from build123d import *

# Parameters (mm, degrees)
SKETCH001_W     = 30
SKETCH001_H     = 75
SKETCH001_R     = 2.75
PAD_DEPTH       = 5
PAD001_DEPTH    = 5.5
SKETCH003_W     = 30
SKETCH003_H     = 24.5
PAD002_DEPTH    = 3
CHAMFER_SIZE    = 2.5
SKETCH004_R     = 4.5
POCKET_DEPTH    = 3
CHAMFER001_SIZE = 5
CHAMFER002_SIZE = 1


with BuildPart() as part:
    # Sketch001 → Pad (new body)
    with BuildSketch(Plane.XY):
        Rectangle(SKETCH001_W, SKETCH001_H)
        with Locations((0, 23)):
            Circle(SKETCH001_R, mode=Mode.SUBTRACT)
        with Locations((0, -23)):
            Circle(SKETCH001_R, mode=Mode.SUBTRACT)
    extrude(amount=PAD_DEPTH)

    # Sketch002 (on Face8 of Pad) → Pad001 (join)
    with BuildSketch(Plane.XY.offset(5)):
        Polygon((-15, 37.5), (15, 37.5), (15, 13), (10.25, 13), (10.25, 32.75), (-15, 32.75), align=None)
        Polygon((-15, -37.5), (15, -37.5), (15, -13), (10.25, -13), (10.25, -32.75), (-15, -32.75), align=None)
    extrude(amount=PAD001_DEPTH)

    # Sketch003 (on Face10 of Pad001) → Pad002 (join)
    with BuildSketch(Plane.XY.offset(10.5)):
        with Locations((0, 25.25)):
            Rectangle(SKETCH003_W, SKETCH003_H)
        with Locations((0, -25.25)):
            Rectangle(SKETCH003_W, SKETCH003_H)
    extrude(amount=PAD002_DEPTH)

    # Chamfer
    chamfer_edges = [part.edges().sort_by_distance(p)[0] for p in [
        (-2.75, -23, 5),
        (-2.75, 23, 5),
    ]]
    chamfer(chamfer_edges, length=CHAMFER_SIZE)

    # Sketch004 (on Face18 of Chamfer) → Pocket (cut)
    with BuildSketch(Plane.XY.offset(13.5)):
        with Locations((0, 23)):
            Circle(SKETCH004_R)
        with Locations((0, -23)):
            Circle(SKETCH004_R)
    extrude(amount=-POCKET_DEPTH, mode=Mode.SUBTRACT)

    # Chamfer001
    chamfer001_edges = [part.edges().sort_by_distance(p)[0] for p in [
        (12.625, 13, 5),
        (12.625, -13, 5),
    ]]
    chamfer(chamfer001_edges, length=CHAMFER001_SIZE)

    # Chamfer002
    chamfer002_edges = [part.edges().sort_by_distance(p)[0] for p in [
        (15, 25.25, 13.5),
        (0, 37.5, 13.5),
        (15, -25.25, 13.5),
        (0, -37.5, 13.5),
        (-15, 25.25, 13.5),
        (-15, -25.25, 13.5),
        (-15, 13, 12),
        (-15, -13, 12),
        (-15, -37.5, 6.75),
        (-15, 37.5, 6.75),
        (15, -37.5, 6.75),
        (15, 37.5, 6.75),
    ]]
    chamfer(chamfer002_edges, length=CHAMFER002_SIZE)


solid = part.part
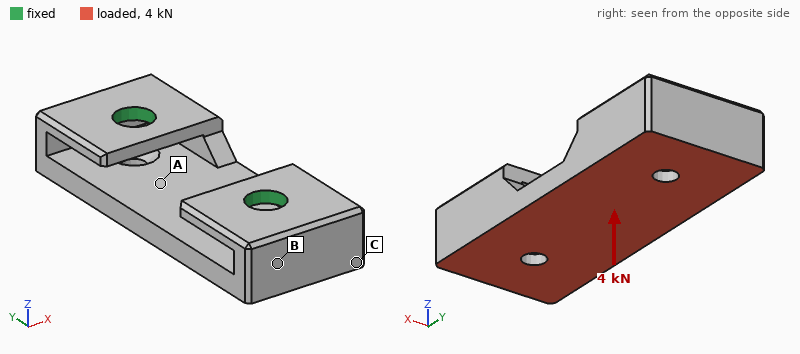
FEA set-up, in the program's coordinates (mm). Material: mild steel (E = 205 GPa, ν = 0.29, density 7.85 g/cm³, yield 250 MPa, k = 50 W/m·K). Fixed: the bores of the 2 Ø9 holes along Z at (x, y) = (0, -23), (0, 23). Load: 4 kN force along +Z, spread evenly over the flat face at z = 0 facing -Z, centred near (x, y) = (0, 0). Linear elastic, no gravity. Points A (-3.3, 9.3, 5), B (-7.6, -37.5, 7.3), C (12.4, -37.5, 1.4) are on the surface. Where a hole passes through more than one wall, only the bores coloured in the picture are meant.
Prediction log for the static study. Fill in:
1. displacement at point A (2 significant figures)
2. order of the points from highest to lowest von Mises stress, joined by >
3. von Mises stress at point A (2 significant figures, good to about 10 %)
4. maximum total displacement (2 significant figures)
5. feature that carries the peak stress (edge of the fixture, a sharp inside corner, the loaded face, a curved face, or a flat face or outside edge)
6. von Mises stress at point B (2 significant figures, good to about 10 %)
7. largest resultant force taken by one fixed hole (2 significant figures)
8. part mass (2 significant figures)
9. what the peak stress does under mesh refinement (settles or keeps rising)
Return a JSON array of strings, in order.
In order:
["45 µm", "B > A > C", "39 MPa", "81 µm", "edge of the fixture", "68 MPa", "2.3 kN", "140 g", "keeps rising"]
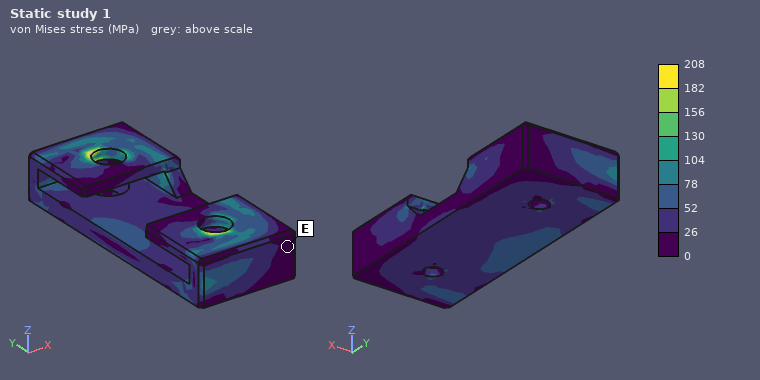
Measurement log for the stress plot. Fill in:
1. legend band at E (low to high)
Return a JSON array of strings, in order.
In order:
["0 to 26 MPa"]
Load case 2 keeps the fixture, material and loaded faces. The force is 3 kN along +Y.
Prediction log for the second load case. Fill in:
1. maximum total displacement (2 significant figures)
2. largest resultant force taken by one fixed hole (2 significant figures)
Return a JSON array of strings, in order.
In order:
["23 µm", "1.6 kN"]
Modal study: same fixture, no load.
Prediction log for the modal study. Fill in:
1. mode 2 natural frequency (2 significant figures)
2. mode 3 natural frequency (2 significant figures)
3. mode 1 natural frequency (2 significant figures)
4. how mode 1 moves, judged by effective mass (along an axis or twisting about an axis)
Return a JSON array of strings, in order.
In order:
["6600 Hz", "6700 Hz", "3900 Hz", "along X"]
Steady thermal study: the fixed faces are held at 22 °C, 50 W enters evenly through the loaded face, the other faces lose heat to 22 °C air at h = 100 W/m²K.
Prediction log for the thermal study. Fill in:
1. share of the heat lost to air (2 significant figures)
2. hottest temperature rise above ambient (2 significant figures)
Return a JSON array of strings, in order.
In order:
["41 %", "59 K"]
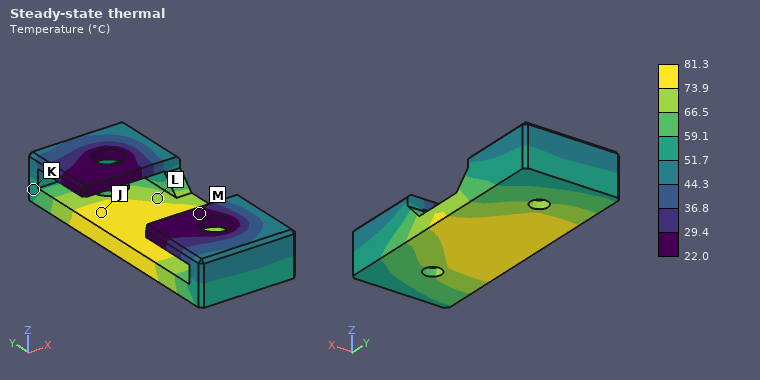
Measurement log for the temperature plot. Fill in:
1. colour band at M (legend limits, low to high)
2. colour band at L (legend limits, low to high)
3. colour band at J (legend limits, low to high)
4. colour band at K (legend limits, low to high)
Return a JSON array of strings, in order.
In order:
["22.0 to 29.4 °C", "66.5 to 73.9 °C", "73.9 to 81.3 °C", "51.7 to 59.1 °C"]
